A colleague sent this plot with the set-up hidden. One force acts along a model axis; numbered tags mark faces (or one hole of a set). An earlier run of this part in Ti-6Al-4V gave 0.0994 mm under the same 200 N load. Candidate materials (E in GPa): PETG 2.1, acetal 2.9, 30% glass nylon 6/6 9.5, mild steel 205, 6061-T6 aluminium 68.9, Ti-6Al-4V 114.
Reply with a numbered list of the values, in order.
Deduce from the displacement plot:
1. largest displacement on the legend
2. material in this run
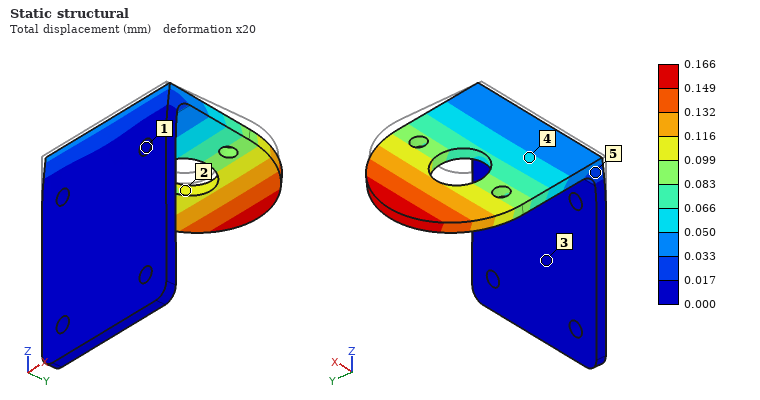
1. 0.166 mm
2. 6061-T6 aluminium
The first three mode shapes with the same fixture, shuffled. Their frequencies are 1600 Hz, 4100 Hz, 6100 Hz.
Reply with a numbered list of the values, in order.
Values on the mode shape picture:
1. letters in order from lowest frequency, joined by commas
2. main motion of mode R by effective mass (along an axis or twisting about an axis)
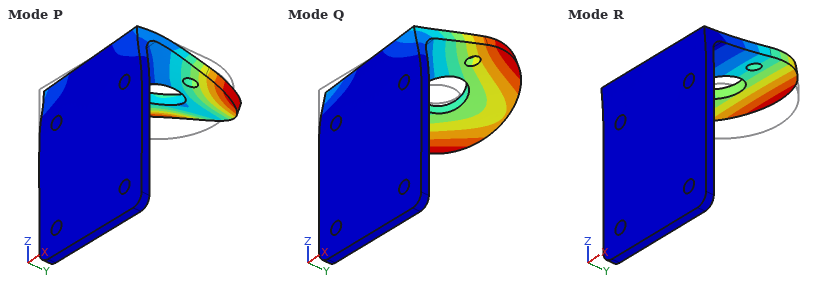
1. R, Q, P
2. along Z
